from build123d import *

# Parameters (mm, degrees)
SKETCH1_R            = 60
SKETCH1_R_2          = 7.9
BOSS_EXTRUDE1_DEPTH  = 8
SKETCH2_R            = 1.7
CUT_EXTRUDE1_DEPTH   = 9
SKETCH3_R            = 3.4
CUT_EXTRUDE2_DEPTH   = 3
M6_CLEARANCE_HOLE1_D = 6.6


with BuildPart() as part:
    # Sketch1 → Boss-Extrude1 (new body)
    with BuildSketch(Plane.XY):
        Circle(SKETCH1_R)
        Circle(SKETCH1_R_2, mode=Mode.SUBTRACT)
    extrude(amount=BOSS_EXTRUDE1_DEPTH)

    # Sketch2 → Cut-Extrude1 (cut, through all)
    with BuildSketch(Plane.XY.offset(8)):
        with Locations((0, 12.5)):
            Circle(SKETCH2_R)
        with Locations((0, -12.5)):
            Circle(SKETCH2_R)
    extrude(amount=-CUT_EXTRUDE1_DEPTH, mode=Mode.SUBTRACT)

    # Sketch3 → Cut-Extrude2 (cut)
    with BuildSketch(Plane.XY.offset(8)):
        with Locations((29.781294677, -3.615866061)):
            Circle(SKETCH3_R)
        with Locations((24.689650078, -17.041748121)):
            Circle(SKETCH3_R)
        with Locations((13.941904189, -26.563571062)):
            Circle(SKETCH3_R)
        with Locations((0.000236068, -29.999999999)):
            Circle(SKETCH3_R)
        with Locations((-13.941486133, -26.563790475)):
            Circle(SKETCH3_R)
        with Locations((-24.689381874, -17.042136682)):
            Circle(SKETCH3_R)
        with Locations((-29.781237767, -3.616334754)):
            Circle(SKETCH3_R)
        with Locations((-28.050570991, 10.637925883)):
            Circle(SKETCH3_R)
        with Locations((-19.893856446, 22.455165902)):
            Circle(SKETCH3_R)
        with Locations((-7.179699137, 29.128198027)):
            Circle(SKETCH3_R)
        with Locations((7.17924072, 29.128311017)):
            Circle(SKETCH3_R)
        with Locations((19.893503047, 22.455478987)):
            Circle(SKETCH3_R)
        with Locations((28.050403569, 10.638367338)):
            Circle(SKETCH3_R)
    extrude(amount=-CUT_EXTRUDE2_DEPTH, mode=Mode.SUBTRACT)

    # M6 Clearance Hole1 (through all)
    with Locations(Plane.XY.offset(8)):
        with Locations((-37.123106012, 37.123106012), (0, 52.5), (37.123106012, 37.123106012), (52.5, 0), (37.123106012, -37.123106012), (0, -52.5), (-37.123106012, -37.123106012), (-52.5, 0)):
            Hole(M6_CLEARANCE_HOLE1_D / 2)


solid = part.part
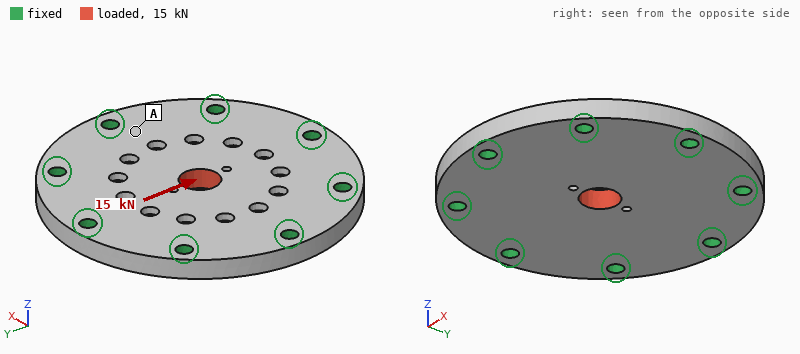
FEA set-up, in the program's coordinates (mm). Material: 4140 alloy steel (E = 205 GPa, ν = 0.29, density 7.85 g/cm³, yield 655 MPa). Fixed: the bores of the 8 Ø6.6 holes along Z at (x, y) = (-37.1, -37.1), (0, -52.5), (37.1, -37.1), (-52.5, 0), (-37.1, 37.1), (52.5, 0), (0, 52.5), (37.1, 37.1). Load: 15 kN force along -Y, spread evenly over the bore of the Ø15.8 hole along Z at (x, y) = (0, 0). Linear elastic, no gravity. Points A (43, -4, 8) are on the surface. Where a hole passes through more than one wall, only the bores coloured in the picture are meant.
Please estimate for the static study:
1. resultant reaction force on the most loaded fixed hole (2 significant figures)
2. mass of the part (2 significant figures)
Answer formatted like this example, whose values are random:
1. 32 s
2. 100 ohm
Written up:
1. 3.1 kN
2. 670 g
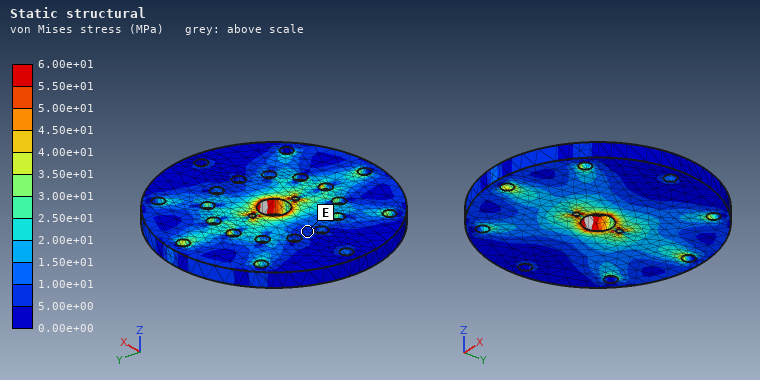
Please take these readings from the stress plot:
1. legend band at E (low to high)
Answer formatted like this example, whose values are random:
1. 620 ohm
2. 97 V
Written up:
1. 5.00e+00 to 1.00e+01 MPa
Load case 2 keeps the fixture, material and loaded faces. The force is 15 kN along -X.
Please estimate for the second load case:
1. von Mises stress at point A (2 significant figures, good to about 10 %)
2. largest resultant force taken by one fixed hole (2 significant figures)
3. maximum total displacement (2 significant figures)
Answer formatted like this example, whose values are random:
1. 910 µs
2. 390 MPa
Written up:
1. 18 MPa
2. 3.1 kN
3. 5.3 µm
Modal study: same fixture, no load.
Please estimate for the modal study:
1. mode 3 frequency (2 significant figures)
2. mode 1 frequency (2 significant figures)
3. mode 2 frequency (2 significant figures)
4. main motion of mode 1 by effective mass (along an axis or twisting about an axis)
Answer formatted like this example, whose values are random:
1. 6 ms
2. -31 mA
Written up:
1. 12 kHz
2. 6300 Hz
3. 12 kHz
4. along Z
